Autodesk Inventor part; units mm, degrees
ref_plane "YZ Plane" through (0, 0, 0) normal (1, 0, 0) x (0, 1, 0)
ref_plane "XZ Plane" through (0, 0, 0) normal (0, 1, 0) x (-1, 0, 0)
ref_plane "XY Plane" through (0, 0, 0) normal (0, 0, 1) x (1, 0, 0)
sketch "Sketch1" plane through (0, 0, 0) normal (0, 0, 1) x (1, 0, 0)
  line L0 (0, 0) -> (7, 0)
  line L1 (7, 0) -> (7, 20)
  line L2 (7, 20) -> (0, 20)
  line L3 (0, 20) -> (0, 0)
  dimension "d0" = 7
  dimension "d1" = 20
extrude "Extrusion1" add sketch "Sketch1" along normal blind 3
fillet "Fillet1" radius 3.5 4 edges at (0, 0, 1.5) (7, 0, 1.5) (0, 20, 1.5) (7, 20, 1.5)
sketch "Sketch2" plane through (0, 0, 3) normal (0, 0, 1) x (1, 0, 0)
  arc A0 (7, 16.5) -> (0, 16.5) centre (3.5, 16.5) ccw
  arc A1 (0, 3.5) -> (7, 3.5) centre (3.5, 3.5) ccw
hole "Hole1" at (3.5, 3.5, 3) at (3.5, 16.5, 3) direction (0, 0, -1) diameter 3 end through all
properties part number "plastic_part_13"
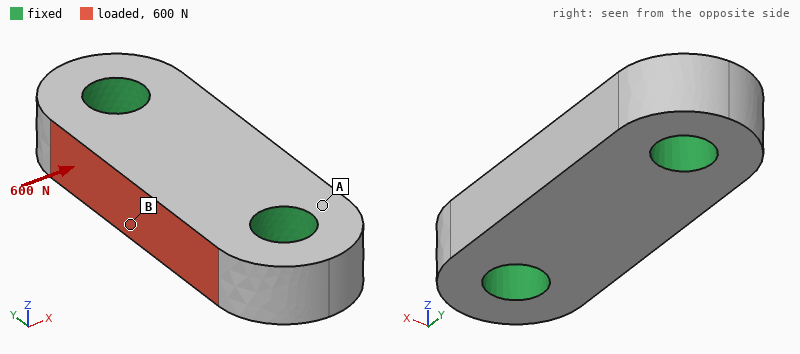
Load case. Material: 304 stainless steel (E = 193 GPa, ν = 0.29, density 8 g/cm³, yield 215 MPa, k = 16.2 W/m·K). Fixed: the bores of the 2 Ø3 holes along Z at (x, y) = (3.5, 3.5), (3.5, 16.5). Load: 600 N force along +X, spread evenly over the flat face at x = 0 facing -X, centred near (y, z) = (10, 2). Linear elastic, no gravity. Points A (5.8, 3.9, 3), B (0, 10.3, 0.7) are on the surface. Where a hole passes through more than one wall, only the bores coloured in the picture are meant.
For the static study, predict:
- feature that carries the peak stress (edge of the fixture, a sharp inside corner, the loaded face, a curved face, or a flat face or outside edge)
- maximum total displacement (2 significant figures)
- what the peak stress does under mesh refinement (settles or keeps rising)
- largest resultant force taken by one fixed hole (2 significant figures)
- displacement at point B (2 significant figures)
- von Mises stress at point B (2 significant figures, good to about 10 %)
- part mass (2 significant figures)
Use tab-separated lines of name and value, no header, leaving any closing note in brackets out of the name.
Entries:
feature that carries the peak stress	edge of the fixture
maximum total displacement	0.94 µm
what the peak stress does under mesh refinement	keeps rising
largest resultant force taken by one fixed hole	300 N
displacement at point B	0.92 µm
von Mises stress at point B	21 MPa
part mass	2.8 g
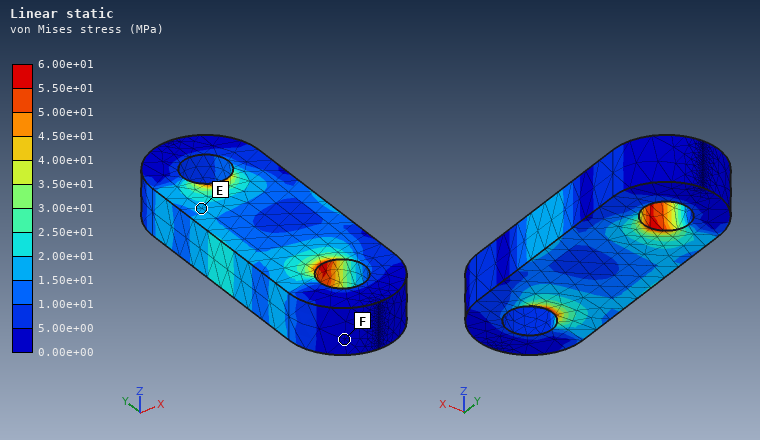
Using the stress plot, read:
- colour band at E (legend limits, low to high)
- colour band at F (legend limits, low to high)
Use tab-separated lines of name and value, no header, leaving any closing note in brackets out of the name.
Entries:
colour band at E	1.50e+01 to 2.00e+01 MPa
colour band at F	0.00e+00 to 5.00e+00 MPa
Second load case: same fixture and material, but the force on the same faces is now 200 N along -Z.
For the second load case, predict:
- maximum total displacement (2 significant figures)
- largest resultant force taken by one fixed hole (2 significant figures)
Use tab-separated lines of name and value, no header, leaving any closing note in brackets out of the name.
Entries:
maximum total displacement	1.6 µm
largest resultant force taken by one fixed hole	100 N
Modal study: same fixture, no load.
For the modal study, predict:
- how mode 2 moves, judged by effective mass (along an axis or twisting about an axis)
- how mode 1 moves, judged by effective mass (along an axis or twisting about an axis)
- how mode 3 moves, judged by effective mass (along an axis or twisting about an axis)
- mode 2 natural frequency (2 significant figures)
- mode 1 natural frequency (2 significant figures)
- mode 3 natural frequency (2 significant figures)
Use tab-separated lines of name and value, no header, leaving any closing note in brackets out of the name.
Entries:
how mode 2 moves, judged by effective mass	twisting about Y
how mode 1 moves, judged by effective mass	along Z
how mode 3 moves, judged by effective mass	along X
mode 2 natural frequency	97 kHz
mode 1 natural frequency	84 kHz
mode 3 natural frequency	100 kHz
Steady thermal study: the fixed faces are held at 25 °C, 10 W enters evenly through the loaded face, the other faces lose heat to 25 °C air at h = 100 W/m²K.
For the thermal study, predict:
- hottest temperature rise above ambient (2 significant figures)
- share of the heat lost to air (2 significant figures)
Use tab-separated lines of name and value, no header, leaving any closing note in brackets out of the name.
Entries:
hottest temperature rise above ambient	73 K
share of the heat lost to air	5.3 %
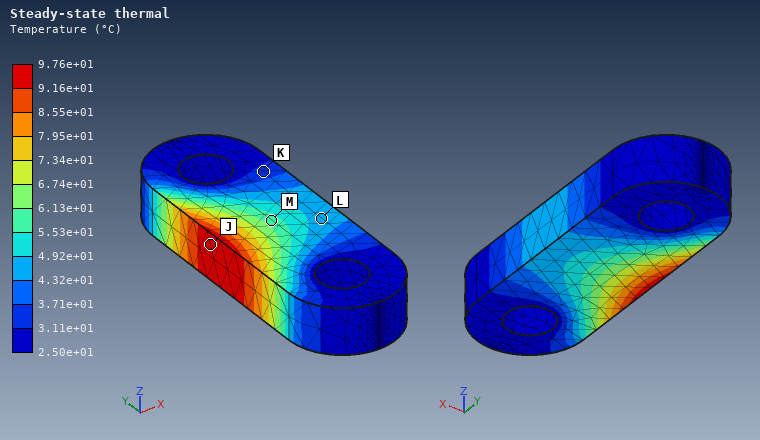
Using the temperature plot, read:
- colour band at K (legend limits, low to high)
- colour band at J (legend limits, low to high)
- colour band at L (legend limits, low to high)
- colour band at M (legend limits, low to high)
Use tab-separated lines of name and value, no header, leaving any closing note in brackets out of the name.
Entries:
colour band at K	3.11e+01 to 3.71e+01 °C
colour band at J	9.16e+01 to 9.76e+01 °C
colour band at L	4.32e+01 to 4.92e+01 °C
colour band at M	5.53e+01 to 6.13e+01 °C
